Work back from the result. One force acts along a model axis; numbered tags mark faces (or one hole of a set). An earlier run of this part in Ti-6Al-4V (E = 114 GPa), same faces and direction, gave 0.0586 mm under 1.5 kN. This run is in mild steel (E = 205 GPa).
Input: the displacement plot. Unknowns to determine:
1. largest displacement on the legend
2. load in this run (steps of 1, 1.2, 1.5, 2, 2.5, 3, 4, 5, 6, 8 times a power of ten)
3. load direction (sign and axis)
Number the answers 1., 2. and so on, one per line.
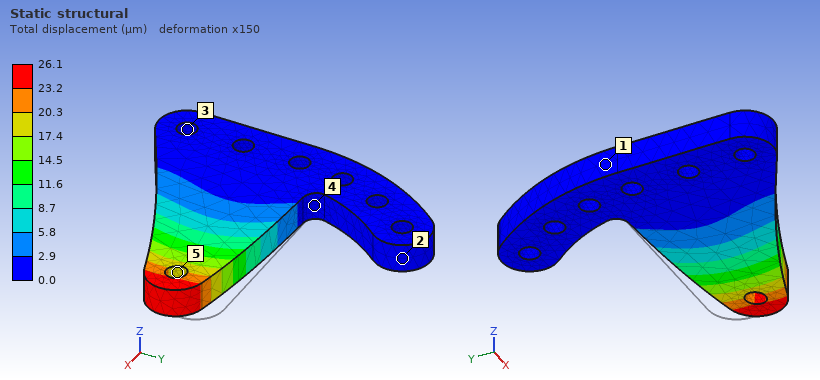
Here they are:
1. 26.1 µm
2. 1.2 kN
3. -Y
